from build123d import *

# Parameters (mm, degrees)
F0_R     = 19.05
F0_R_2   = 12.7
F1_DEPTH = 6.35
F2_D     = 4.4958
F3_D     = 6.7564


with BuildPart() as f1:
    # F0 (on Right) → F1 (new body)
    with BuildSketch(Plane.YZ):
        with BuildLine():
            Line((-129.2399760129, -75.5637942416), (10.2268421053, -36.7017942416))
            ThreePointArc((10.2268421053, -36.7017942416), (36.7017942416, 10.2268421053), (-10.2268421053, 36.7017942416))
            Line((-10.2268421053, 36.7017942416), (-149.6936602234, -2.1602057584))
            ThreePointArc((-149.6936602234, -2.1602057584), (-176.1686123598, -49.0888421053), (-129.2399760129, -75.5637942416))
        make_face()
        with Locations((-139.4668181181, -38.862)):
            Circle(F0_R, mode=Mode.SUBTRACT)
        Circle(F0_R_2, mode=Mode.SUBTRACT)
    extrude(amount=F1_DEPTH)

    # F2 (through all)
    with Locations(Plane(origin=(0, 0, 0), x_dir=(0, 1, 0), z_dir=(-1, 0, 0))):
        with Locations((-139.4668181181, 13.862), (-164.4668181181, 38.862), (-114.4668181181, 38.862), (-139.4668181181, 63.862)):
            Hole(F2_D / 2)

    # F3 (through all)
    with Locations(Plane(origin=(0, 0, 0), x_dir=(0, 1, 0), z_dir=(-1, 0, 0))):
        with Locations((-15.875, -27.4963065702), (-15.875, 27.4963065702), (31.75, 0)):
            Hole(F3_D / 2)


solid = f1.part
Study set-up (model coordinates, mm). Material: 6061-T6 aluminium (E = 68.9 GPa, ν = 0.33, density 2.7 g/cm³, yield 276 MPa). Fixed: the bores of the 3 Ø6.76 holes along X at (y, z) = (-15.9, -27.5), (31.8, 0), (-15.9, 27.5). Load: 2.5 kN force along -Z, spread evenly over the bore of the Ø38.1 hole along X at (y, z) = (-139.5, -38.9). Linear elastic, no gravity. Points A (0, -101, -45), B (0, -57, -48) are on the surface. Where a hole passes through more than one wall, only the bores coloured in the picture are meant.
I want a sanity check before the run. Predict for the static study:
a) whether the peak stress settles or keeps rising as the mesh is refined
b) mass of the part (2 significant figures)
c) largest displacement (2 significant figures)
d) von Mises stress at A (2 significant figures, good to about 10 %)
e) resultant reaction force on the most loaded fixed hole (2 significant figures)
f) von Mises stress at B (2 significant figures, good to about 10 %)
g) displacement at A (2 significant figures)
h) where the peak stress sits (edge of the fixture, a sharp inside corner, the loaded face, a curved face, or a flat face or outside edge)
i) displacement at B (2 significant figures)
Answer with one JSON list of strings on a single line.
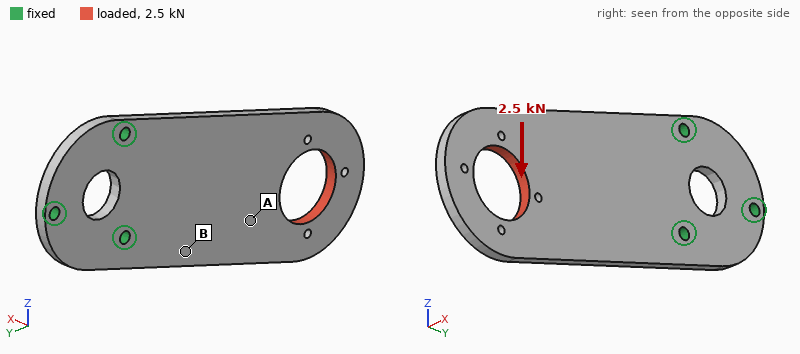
["keeps rising", "240 g", "0.22 mm", "9.9 MPa", "5.6 kN", "23 MPa", "0.094 mm", "edge of the fixture", "0.046 mm"]
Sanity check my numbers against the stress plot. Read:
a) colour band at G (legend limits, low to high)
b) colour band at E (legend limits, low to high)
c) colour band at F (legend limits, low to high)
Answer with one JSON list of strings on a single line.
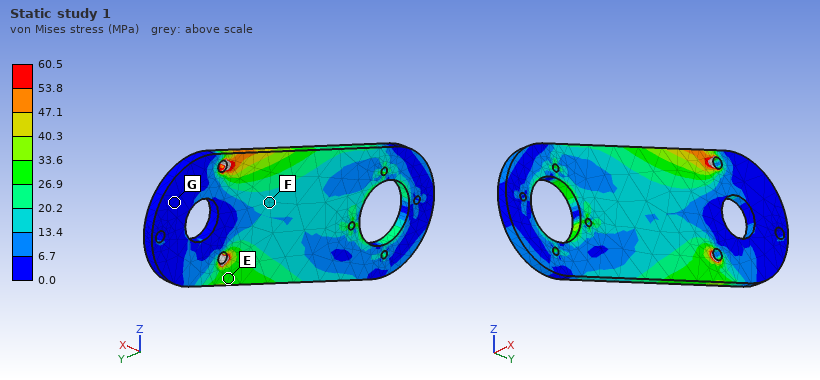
["0.0 to 6.7 MPa", "26.9 to 33.6 MPa", "13.4 to 20.2 MPa"]
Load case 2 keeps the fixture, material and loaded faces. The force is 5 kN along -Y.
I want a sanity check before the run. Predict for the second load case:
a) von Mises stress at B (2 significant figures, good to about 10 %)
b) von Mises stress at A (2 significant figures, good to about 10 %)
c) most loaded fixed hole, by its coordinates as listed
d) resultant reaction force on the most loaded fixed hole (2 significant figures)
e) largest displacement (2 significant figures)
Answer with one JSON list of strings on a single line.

["24 MPa", "11 MPa", "(-15.9, -27.5)", "5.4 kN", "0.12 mm"]
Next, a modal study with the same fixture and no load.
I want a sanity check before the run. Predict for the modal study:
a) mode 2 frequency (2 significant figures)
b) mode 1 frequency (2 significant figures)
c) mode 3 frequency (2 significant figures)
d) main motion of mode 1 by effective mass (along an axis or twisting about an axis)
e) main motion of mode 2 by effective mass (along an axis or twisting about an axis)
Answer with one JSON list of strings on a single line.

["930 Hz", "230 Hz", "1200 Hz", "along X", "twisting about Y"]
